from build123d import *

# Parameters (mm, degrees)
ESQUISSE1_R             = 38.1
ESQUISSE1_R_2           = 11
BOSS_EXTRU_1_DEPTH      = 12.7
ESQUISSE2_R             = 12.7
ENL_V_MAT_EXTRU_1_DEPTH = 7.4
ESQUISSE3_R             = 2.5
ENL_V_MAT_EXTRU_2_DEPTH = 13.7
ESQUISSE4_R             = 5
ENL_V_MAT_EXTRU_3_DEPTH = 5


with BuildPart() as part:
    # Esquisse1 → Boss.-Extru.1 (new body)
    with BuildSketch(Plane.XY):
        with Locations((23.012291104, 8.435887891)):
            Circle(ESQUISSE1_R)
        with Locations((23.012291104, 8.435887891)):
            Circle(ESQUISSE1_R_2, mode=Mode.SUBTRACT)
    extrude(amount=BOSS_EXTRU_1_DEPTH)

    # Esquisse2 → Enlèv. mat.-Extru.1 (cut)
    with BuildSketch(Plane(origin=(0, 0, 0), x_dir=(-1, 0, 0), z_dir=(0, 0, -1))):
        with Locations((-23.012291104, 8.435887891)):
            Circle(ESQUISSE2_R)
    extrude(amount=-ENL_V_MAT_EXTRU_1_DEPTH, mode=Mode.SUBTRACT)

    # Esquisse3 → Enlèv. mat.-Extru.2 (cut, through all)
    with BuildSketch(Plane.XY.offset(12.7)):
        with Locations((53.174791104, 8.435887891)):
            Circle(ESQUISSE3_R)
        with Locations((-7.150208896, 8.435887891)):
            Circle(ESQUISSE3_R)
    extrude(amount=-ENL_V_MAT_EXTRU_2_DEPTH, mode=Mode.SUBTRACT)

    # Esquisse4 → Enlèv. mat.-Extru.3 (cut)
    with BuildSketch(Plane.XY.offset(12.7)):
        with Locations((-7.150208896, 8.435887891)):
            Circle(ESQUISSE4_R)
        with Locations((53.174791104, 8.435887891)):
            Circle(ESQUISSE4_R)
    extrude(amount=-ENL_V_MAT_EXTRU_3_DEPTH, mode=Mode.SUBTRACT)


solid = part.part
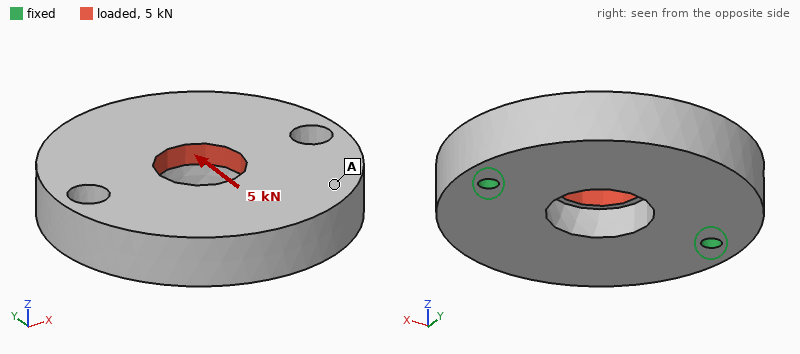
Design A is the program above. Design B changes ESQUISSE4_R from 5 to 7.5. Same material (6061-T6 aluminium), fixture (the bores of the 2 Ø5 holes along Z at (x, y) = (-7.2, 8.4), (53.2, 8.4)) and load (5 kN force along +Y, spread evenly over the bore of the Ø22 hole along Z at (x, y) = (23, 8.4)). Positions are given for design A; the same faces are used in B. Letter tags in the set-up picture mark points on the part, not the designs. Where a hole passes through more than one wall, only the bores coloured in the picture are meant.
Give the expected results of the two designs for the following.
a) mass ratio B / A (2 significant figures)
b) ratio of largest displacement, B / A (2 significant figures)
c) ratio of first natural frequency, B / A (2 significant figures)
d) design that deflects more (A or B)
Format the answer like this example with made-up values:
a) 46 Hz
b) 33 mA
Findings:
a) 0.98
b) 1.2
c) 0.94
d) B
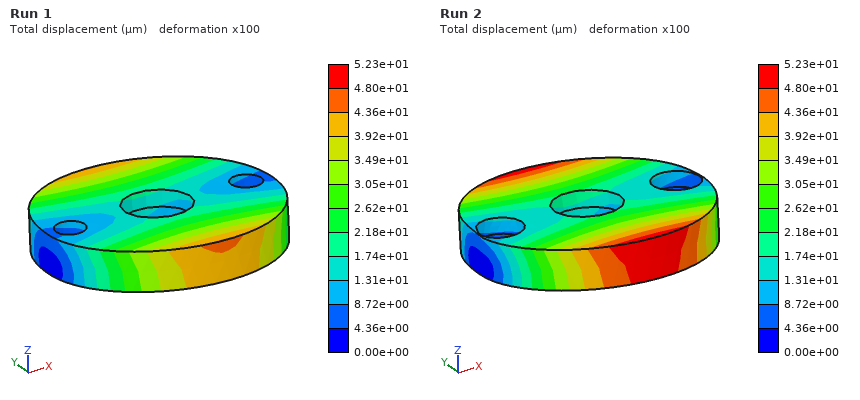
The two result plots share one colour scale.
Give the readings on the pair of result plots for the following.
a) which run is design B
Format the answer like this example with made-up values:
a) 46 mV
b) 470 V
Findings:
a) Run 2
